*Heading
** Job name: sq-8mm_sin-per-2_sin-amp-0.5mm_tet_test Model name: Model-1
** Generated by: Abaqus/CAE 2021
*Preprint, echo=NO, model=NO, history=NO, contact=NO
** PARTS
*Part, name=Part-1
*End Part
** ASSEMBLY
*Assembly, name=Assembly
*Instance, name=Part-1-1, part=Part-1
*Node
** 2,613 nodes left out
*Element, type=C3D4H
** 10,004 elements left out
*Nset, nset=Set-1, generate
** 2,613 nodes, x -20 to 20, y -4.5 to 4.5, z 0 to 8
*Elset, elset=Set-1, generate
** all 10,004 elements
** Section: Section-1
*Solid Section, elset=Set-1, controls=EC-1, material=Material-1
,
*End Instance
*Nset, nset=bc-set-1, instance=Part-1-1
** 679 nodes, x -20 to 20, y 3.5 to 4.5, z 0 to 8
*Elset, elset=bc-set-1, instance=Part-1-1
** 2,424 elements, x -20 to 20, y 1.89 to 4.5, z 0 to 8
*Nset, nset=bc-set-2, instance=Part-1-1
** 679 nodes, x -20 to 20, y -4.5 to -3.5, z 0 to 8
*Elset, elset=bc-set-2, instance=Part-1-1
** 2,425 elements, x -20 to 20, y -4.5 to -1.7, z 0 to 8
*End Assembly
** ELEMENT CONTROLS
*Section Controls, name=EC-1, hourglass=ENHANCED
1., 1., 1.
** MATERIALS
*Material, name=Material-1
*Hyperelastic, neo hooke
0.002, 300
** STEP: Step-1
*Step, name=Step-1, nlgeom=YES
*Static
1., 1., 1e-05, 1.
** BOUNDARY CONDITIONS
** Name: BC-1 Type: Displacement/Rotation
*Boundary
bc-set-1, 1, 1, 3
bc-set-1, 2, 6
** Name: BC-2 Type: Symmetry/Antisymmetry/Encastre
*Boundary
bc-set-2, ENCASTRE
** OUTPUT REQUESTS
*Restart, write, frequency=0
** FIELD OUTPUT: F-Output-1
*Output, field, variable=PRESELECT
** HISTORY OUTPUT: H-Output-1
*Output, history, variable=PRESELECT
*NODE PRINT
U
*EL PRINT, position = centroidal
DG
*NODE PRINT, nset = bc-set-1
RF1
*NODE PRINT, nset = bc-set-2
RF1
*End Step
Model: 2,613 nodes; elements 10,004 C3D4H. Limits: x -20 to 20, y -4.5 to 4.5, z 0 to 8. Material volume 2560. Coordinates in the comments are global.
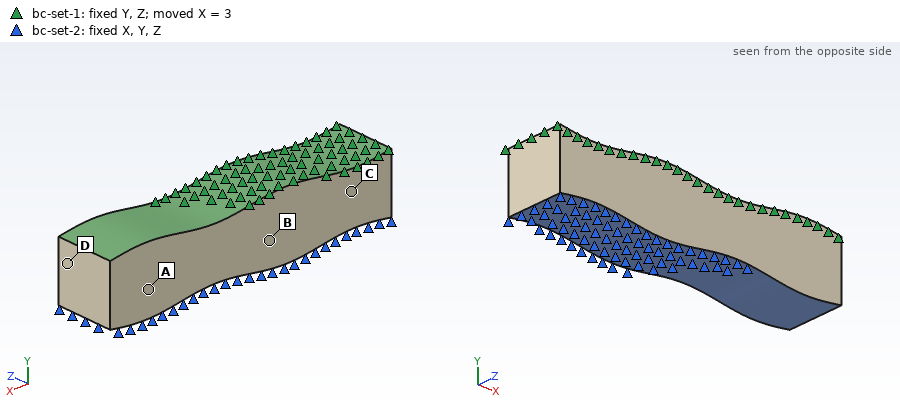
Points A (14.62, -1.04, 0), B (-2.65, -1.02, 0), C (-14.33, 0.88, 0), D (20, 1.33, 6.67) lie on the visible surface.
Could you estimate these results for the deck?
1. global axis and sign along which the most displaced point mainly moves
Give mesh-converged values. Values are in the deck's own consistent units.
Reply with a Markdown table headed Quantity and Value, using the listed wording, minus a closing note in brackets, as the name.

| Quantity | Value |
|---|---|
| global axis and sign along which the most displaced point mainly moves | +X |
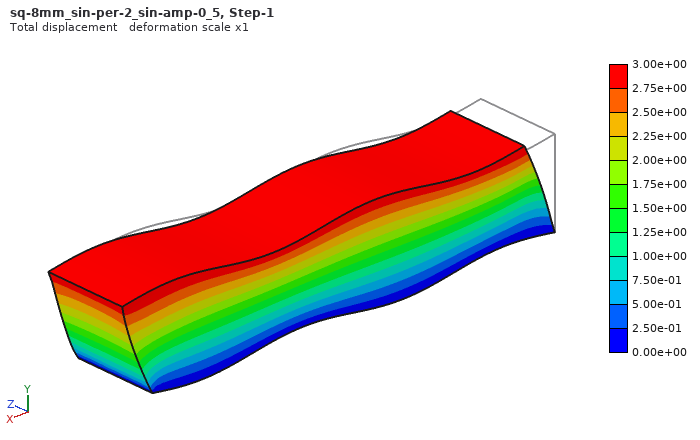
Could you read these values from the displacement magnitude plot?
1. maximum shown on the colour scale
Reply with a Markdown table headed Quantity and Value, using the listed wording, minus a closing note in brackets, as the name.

| Quantity | Value |
|---|---|
| maximum shown on the colour scale | 3.00e+00 |
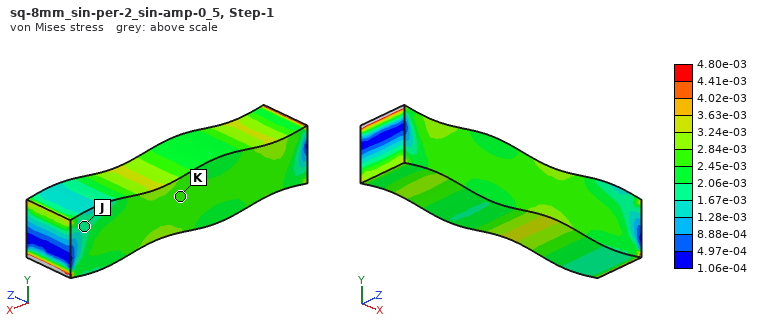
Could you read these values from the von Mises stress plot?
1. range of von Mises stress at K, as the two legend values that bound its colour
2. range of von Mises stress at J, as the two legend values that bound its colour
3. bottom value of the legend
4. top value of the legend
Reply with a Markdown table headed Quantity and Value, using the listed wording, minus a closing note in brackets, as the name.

| Quantity | Value |
|---|---|
| range of von Mises stress at K, as the two legend values that bound its colour | 2.45e-03 to 2.84e-03 |
| range of von Mises stress at J, as the two legend values that bound its colour | 1.67e-03 to 2.06e-03 |
| bottom value of the legend | 1.06e-04 |
| top value of the legend | 4.80e-03 |
